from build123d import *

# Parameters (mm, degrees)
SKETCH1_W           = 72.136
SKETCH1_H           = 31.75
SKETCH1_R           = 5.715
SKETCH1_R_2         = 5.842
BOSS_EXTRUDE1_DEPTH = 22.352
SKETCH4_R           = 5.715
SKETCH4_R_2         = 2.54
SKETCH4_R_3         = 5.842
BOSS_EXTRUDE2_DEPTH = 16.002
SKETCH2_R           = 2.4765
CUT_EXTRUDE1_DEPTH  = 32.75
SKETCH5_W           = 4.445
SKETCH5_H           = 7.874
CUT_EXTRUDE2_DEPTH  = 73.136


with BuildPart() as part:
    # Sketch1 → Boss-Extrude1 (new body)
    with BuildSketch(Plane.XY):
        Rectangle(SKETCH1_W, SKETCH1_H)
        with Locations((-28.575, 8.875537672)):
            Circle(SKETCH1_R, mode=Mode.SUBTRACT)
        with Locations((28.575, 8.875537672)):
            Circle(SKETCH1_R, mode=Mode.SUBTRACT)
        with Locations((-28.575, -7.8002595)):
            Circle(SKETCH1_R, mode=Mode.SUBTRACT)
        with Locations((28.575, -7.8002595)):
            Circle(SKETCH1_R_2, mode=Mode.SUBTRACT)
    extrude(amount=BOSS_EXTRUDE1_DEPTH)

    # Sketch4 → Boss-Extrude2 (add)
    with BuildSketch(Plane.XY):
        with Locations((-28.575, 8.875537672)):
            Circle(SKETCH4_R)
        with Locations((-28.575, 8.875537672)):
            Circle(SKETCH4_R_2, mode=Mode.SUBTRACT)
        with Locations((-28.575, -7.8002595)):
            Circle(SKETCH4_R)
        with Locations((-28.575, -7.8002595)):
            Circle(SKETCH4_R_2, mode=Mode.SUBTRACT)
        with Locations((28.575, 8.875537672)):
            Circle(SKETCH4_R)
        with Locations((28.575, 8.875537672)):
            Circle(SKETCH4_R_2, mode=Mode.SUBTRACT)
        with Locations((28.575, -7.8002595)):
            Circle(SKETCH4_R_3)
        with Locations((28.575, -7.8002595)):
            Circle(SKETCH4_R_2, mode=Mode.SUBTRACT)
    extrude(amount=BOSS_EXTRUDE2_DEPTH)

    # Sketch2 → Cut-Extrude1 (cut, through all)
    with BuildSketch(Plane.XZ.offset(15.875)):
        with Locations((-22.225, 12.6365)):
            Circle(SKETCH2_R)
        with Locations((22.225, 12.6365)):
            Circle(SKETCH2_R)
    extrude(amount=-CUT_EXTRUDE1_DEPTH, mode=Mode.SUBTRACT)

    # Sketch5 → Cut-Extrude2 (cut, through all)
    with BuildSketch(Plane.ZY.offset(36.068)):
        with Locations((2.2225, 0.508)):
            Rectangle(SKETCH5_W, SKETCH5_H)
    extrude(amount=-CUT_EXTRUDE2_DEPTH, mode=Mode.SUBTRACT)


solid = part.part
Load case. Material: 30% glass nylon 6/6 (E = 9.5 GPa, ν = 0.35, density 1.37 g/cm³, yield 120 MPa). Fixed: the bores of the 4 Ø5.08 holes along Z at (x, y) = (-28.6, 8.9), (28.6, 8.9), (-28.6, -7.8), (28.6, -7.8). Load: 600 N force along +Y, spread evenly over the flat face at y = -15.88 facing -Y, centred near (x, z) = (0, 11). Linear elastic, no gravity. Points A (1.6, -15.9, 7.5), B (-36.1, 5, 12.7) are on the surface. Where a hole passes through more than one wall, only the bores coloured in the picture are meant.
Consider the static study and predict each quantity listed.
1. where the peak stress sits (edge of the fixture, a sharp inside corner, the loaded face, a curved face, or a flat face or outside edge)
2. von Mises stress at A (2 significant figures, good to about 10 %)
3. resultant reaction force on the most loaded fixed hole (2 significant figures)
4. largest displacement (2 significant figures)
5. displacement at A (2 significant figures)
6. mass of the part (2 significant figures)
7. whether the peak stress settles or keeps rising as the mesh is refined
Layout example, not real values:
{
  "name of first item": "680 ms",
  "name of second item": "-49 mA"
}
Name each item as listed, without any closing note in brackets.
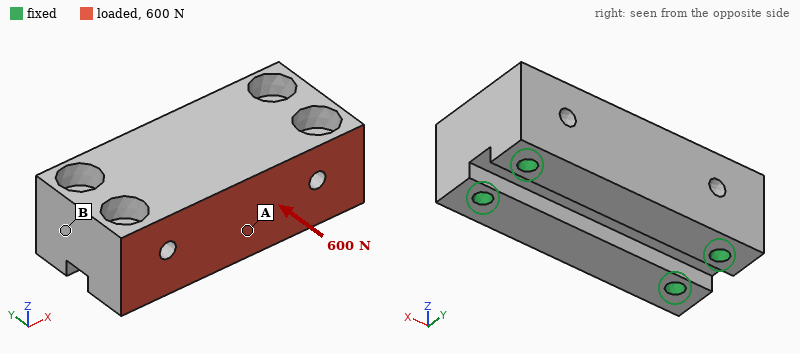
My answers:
{
  "where the peak stress sits": "edge of the fixture",
  "von Mises stress at A": "0.62 MPa",
  "resultant reaction force on the most loaded fixed hole": "200 N",
  "largest displacement": "3.7 µm",
  "displacement at A": "3.4 µm",
  "mass of the part": "60 g",
  "whether the peak stress settles or keeps rising as the mesh is refined": "keeps rising"
}
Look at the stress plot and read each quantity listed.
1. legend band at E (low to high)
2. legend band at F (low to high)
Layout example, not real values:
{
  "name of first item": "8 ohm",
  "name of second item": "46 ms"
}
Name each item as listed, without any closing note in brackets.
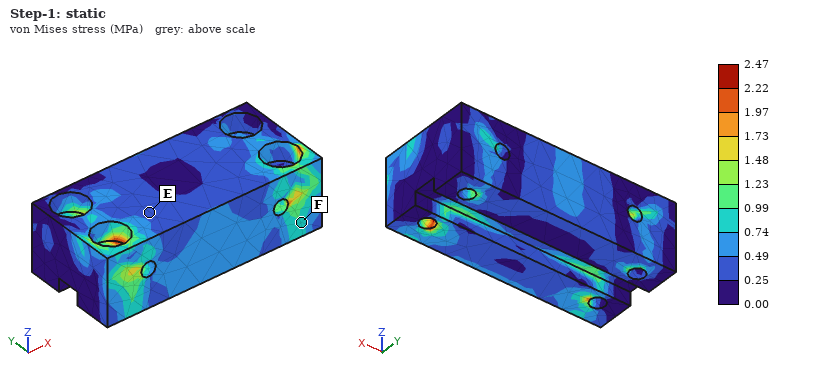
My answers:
{
  "legend band at E": "0.25 to 0.49 MPa",
  "legend band at F": "0.74 to 0.99 MPa"
}
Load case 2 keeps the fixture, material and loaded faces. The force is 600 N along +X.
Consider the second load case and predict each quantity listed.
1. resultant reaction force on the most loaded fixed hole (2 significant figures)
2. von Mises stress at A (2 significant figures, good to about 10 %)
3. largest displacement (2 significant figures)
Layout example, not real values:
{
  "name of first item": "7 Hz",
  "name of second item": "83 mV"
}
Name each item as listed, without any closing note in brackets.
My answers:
{
  "resultant reaction force on the most loaded fixed hole": "250 N",
  "von Mises stress at A": "0.70 MPa",
  "largest displacement": "3.7 µm"
}
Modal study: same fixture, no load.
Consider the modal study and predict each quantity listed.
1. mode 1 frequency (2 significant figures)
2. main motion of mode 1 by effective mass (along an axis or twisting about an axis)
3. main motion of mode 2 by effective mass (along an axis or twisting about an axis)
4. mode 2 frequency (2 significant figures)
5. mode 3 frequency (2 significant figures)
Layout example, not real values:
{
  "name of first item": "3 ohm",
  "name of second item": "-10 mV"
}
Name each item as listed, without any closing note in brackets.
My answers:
{
  "mode 1 frequency": "8700 Hz",
  "main motion of mode 1 by effective mass": "along Z",
  "main motion of mode 2 by effective mass": "along Y",
  "mode 2 frequency": "9400 Hz",
  "mode 3 frequency": "10 kHz"
}
